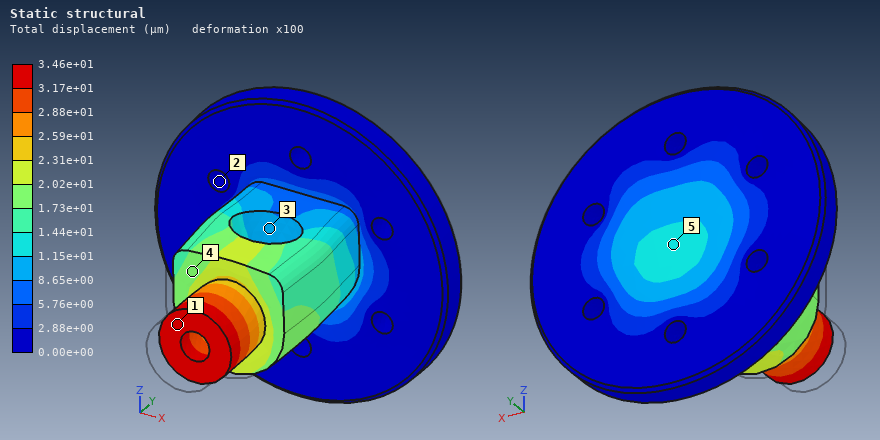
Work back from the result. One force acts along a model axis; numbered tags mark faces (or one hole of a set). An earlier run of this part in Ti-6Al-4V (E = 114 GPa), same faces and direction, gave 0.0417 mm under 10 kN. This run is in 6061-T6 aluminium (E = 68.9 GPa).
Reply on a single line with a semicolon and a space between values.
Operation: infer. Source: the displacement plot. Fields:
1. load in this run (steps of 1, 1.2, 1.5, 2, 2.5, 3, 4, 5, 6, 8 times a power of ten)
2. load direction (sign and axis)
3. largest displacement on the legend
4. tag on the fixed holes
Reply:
5 kN; +Y; 3.46e+01 µm; 2
